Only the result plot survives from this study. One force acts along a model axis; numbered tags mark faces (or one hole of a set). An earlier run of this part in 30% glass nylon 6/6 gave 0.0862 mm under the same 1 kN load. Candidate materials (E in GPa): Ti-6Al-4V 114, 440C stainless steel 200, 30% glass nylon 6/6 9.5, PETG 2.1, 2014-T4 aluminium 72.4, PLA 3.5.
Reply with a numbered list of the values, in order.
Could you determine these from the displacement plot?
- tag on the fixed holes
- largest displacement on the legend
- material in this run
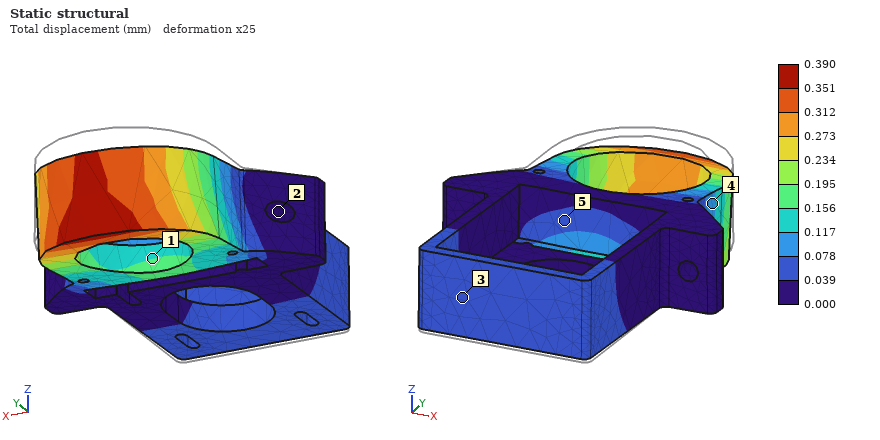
1. 2
2. 0.390 mm
3. PETG
